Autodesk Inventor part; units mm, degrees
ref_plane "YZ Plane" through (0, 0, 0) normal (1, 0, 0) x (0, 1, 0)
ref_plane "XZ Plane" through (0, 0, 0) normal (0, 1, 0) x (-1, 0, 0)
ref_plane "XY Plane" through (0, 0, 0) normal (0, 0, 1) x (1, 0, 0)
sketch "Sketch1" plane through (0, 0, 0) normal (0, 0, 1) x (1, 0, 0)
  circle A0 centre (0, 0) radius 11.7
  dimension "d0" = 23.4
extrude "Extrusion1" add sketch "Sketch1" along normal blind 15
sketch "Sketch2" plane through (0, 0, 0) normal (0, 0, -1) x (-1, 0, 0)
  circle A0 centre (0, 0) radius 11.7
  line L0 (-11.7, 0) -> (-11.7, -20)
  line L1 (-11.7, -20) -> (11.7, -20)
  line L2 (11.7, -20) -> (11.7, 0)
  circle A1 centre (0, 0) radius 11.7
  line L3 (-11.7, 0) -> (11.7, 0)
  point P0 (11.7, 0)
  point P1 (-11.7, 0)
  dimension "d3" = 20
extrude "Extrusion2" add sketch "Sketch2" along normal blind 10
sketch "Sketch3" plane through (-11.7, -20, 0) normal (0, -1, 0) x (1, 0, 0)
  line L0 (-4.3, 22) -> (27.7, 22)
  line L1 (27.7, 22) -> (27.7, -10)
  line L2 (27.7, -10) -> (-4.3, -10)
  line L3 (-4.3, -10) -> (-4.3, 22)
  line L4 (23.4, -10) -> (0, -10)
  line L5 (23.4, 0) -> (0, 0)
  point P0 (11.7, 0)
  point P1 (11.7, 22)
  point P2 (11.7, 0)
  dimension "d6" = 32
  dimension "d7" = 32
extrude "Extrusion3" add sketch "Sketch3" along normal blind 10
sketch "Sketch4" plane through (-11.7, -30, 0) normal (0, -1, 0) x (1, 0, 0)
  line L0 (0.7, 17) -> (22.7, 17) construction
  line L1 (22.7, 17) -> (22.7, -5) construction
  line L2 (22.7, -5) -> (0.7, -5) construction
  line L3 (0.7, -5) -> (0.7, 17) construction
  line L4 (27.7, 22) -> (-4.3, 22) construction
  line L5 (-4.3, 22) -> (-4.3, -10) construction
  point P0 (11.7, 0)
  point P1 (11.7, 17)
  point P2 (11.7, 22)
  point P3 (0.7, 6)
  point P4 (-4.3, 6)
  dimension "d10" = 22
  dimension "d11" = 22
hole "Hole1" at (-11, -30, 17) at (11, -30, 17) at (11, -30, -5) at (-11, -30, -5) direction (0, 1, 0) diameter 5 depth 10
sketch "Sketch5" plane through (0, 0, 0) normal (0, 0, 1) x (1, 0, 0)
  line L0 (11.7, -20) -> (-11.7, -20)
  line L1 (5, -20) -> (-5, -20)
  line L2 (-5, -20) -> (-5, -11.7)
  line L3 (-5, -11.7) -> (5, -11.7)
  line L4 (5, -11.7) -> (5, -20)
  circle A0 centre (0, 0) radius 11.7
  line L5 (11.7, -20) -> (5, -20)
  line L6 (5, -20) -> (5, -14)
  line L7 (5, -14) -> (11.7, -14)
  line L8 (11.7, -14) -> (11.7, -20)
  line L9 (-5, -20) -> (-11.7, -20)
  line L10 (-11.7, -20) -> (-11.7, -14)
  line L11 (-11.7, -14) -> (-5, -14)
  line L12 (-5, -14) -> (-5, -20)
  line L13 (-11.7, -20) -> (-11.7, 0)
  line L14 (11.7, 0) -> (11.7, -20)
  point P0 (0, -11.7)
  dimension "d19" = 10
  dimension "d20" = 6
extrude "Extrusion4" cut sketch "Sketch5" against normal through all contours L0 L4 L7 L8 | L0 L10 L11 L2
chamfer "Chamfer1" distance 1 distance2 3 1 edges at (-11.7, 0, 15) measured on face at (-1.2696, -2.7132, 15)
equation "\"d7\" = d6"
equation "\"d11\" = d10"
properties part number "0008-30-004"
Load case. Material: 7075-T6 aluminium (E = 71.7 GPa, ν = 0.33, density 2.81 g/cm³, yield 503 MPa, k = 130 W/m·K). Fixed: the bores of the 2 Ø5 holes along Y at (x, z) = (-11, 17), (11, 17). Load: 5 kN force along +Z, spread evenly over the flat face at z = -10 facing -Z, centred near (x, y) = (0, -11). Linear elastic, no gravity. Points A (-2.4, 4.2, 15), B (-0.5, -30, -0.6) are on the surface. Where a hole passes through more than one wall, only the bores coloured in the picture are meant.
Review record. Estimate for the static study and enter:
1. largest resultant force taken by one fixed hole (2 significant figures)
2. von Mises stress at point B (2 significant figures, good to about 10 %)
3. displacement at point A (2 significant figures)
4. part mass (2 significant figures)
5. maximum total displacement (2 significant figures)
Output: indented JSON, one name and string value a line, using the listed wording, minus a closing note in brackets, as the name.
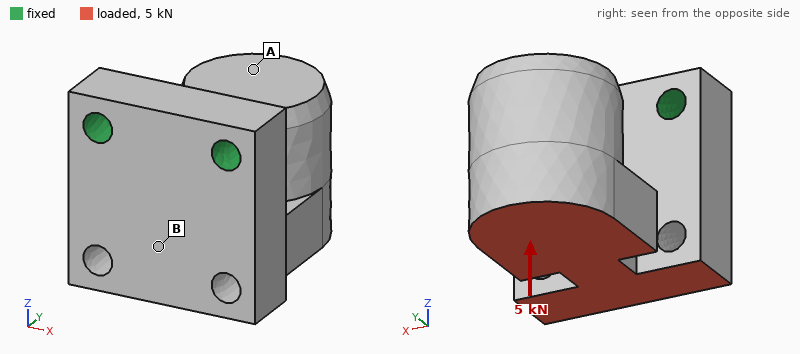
{
  "largest resultant force taken by one fixed hole": "2.6 kN",
  "von Mises stress at point B": "120 MPa",
  "displacement at point A": "0.52 mm",
  "part mass": "61 g",
  "maximum total displacement": "0.62 mm"
}
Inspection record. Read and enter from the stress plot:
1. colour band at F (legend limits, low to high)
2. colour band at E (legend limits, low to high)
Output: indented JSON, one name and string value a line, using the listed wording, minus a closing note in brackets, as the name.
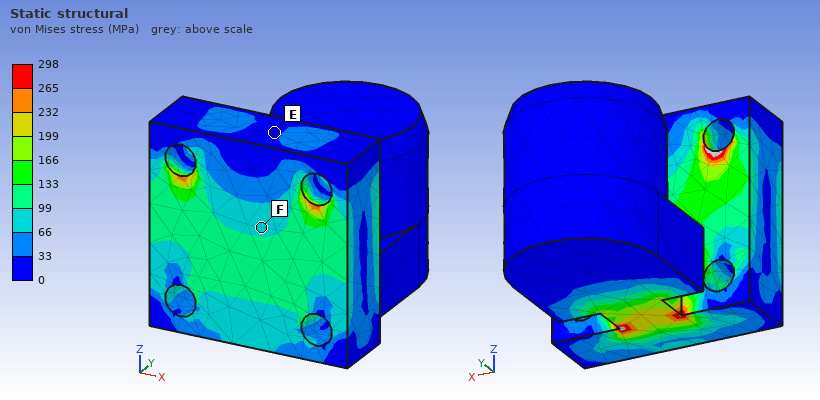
{
  "colour band at F": "66 to 99 MPa",
  "colour band at E": "0 to 33 MPa"
}
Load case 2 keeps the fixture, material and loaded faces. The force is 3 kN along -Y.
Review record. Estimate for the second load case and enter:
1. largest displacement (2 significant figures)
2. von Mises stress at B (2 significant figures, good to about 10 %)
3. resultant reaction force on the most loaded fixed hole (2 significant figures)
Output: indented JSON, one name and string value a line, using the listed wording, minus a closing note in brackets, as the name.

{
  "largest displacement": "0.31 mm",
  "von Mises stress at B": "62 MPa",
  "resultant reaction force on the most loaded fixed hole": "1.5 kN"
}
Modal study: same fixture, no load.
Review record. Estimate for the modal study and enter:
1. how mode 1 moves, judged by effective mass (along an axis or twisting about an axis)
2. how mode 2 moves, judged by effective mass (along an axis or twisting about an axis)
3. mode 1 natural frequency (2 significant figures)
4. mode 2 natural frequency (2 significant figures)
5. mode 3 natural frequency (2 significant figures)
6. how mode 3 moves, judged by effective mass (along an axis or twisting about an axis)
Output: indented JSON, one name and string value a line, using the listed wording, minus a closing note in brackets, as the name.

{
  "how mode 1 moves, judged by effective mass": "along Z",
  "how mode 2 moves, judged by effective mass": "along X",
  "mode 1 natural frequency": "2200 Hz",
  "mode 2 natural frequency": "2400 Hz",
  "mode 3 natural frequency": "5400 Hz",
  "how mode 3 moves, judged by effective mass": "along Y"
}
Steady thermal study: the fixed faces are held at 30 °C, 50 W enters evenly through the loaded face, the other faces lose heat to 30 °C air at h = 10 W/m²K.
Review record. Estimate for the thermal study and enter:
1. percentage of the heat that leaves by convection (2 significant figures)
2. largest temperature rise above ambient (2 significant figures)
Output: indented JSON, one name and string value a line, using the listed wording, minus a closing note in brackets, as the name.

{
  "percentage of the heat that leaves by convection": "3.5 %",
  "largest temperature rise above ambient": "60 K"
}
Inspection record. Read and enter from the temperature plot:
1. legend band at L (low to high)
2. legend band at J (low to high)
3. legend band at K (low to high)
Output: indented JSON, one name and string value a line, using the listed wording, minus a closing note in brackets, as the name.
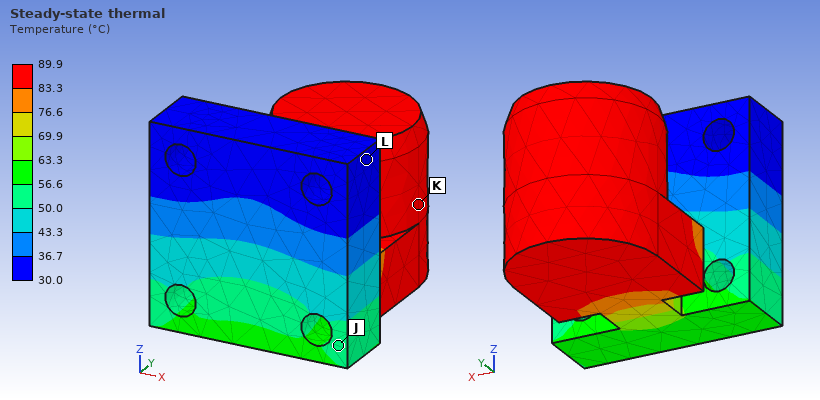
{
  "legend band at L": "30.0 to 36.7 °C",
  "legend band at J": "50.0 to 56.6 °C",
  "legend band at K": "83.3 to 89.9 °C"
}
